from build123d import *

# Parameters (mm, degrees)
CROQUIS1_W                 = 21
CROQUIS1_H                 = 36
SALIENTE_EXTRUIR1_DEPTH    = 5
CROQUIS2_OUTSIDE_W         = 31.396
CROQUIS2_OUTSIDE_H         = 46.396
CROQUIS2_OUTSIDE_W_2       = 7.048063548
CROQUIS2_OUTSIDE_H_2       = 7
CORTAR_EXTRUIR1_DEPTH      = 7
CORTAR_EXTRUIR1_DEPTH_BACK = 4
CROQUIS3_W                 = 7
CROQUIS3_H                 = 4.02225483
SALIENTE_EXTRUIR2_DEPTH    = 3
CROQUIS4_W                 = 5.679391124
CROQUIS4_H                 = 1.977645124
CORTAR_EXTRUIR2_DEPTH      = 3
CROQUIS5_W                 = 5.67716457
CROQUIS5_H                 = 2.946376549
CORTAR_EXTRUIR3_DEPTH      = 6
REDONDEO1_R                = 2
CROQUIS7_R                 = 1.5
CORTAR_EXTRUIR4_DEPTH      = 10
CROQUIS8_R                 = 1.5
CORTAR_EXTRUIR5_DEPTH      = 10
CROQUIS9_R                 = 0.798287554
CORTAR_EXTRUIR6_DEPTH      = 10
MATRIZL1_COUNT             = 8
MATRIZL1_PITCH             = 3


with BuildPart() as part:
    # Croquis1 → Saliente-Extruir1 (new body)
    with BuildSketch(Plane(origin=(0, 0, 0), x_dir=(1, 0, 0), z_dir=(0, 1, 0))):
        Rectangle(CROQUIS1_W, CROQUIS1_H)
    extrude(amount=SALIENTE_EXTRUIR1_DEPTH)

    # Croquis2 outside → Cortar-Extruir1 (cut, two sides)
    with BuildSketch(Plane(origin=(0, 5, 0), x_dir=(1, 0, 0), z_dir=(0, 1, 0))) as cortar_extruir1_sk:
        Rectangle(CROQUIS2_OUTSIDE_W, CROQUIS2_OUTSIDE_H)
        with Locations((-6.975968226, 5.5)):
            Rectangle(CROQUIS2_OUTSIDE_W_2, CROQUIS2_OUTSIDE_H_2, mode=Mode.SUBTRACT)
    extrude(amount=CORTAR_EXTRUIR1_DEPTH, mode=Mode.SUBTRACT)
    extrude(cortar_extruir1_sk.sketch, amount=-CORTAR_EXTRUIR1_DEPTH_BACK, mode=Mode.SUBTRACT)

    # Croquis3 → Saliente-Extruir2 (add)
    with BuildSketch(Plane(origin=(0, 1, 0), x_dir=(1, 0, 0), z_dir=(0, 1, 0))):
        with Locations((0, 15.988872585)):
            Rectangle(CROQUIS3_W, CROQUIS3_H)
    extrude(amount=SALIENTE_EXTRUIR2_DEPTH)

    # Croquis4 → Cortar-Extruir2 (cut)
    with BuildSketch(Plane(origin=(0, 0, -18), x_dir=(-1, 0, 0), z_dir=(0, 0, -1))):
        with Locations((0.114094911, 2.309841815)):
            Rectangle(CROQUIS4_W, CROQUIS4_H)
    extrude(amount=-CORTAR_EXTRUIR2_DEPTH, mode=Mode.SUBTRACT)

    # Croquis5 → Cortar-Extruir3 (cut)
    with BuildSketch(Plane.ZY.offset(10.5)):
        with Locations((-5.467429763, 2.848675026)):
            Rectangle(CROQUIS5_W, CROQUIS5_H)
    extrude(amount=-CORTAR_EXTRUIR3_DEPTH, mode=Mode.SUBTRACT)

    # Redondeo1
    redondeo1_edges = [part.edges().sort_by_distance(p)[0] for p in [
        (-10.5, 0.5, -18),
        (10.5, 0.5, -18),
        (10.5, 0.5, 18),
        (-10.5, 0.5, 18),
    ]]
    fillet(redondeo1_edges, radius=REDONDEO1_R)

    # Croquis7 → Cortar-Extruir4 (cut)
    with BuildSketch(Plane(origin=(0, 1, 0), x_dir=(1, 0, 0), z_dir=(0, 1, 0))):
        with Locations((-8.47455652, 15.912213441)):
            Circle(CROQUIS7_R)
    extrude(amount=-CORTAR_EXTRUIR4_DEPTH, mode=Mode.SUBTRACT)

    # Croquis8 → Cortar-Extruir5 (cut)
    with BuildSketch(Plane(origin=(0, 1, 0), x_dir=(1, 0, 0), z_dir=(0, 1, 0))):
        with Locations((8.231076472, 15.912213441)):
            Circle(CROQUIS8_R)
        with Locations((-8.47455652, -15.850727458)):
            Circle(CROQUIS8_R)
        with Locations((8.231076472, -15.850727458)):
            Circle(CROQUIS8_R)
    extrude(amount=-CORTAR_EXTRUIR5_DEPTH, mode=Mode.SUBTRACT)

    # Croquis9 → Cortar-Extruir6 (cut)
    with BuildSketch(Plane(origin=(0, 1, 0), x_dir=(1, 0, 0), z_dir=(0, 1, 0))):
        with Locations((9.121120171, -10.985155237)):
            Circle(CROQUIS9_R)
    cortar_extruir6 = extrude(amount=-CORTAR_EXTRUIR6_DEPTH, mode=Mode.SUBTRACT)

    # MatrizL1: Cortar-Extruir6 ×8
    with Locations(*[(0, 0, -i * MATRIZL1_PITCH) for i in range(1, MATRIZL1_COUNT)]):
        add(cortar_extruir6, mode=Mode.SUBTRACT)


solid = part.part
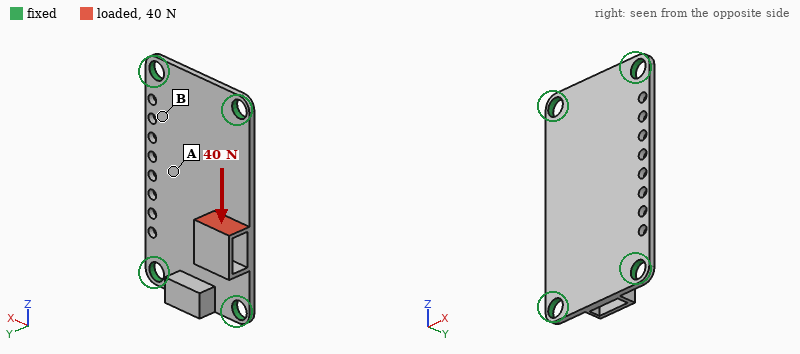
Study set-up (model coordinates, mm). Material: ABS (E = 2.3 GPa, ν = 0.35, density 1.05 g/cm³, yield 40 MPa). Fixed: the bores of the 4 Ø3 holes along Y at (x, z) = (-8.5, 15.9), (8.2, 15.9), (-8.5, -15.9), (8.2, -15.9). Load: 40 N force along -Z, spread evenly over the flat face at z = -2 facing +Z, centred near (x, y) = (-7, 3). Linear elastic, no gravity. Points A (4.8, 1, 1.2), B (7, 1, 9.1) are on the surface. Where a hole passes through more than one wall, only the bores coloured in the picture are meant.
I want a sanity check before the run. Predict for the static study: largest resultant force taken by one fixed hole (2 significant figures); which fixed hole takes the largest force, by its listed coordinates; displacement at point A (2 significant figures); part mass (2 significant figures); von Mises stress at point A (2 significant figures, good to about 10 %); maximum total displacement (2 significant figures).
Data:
20 N
(-8.5, -15.9)
0.18 mm
0.90 g
4.5 MPa
0.43 mm
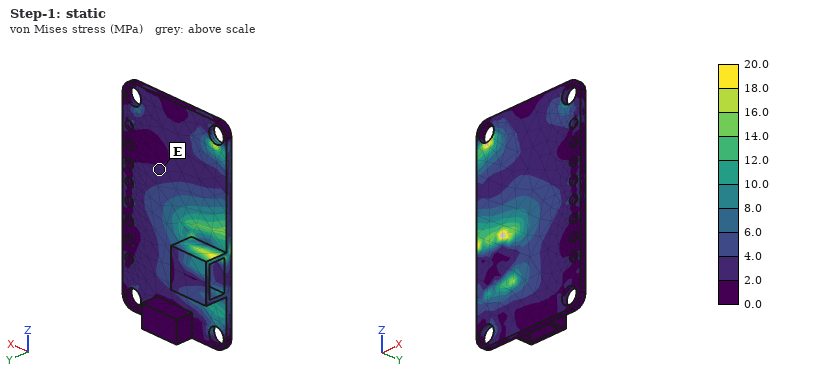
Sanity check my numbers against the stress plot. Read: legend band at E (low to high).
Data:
2.0 to 4.0 MPa
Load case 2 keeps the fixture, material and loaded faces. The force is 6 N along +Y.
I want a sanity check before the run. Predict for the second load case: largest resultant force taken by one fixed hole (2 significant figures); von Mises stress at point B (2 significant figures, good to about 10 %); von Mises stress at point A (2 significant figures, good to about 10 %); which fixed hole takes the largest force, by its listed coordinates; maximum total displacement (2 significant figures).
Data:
3.8 N
1.1 MPa
2.6 MPa
(-8.5, -15.9)
0.34 mm
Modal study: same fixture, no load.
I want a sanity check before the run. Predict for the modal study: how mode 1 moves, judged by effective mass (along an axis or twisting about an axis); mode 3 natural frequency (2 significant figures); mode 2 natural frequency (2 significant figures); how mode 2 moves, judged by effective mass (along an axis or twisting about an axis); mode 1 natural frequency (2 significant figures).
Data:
along Y
4200 Hz
2300 Hz
twisting about Z
1500 Hz
